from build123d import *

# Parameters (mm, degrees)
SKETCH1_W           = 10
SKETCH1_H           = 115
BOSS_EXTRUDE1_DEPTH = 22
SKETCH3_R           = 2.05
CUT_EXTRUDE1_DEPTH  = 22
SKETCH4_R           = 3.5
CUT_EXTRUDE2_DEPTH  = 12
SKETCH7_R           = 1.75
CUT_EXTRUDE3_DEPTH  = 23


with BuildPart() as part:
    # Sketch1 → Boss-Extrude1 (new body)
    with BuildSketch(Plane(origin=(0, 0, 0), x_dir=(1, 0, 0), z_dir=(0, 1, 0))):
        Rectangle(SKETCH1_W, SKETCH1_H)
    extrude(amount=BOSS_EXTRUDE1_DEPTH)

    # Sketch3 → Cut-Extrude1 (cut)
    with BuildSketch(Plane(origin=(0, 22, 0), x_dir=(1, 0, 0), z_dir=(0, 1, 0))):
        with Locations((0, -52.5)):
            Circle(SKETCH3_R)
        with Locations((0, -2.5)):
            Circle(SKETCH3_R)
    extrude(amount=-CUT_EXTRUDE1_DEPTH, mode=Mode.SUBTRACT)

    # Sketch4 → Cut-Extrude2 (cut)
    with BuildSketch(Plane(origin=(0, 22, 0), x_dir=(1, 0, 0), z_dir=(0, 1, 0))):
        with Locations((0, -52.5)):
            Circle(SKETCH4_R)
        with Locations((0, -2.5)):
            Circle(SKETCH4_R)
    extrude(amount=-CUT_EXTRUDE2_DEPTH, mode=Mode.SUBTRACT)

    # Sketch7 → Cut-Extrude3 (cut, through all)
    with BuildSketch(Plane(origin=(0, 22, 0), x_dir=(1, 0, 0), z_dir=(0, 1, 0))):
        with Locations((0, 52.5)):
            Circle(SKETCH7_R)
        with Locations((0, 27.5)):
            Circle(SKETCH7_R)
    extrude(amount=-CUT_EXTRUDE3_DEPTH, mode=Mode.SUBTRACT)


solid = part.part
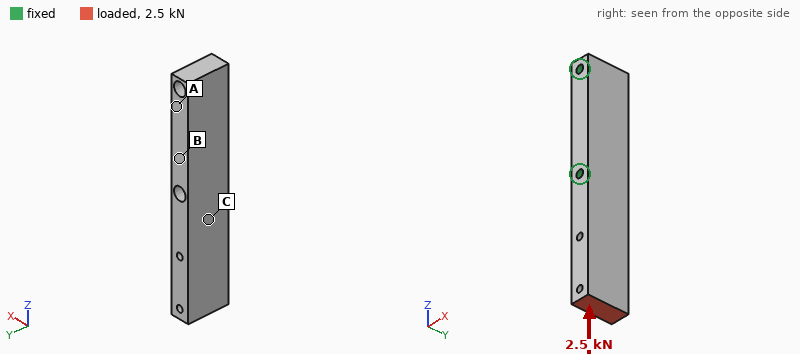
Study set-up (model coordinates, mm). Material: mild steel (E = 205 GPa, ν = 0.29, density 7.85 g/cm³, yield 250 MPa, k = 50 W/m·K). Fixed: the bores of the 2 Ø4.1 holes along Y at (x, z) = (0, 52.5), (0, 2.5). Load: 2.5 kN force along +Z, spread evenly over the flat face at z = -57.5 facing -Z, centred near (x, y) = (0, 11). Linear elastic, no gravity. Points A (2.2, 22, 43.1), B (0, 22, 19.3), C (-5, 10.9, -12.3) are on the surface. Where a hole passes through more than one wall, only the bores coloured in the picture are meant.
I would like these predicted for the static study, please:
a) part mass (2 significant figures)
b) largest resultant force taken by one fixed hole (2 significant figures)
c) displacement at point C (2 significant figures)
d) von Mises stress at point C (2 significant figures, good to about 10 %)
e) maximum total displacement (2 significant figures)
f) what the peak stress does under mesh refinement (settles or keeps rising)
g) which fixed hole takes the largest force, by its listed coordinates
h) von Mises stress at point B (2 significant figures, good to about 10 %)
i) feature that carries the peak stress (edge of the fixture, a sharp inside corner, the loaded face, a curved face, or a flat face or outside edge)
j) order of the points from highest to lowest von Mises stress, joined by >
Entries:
190 g
2.1 kN
2.5 µm
12 MPa
10 µm
keeps rising
(0, 2.5)
6.9 MPa
edge of the fixture
C > B > A
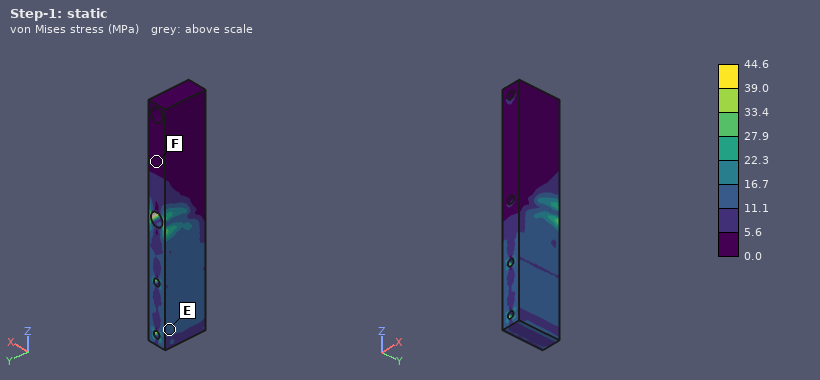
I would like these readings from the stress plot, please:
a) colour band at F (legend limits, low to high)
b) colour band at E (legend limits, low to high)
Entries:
0.0 to 5.6 MPa
11.1 to 16.7 MPa
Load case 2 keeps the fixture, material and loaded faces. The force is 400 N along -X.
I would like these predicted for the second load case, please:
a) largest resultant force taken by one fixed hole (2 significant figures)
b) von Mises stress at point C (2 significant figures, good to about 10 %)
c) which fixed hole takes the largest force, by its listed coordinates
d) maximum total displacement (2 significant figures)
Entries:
620 N
49 MPa
(0, 2.5)
0.10 mm
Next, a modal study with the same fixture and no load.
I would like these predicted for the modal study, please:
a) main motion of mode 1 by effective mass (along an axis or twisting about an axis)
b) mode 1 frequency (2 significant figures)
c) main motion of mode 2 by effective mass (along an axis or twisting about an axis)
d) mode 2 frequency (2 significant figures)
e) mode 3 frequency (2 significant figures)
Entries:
along X
2000 Hz
along Y
3500 Hz
8100 Hz
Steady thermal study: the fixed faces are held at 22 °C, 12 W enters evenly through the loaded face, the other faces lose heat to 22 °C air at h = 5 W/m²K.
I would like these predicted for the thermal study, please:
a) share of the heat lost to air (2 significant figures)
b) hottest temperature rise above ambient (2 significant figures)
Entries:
7.0 %
72 K
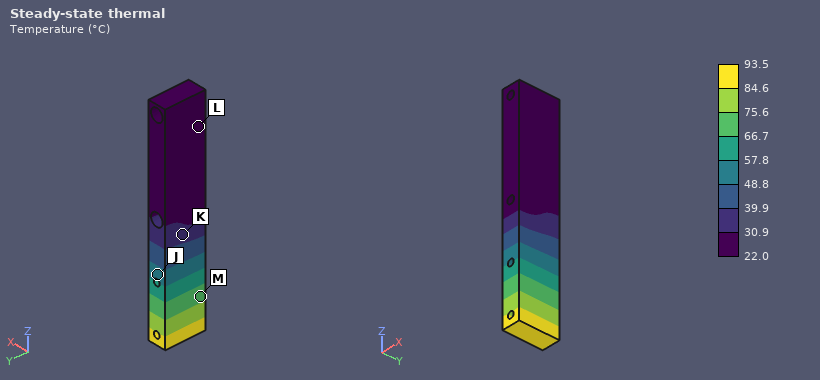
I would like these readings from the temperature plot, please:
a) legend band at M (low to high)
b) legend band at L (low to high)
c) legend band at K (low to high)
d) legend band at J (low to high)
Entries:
66.7 to 75.6 °C
22.0 to 30.9 °C
30.9 to 39.9 °C
48.8 to 57.8 °C
